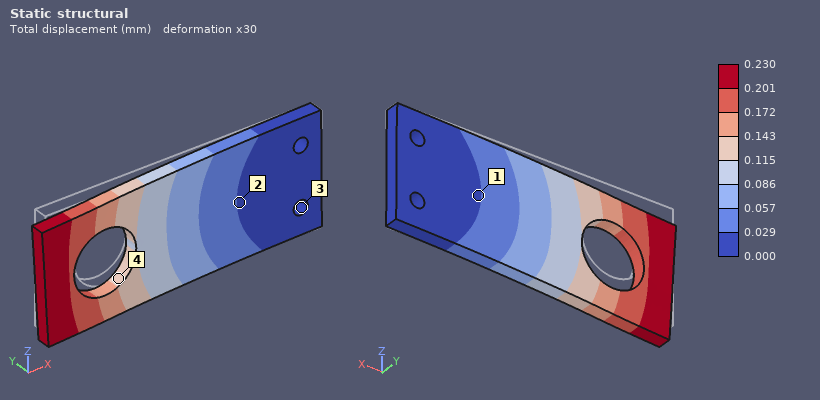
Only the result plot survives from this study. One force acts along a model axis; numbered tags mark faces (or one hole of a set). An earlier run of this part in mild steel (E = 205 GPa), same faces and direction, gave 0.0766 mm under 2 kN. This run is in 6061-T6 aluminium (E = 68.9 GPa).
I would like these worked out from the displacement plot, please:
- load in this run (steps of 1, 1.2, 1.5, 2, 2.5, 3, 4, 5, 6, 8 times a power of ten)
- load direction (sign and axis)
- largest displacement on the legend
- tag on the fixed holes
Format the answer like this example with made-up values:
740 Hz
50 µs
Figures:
2 kN
-Z
0.230 mm
3
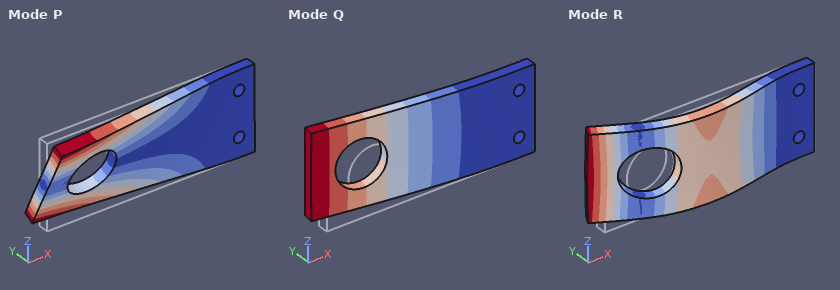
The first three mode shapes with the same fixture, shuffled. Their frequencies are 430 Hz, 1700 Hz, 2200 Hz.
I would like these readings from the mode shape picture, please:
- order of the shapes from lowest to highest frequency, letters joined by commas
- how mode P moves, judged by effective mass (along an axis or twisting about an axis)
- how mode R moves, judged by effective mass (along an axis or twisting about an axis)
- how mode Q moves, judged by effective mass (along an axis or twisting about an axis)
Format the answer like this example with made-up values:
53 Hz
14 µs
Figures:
Q, P, R
twisting about X
along Y
along Y
